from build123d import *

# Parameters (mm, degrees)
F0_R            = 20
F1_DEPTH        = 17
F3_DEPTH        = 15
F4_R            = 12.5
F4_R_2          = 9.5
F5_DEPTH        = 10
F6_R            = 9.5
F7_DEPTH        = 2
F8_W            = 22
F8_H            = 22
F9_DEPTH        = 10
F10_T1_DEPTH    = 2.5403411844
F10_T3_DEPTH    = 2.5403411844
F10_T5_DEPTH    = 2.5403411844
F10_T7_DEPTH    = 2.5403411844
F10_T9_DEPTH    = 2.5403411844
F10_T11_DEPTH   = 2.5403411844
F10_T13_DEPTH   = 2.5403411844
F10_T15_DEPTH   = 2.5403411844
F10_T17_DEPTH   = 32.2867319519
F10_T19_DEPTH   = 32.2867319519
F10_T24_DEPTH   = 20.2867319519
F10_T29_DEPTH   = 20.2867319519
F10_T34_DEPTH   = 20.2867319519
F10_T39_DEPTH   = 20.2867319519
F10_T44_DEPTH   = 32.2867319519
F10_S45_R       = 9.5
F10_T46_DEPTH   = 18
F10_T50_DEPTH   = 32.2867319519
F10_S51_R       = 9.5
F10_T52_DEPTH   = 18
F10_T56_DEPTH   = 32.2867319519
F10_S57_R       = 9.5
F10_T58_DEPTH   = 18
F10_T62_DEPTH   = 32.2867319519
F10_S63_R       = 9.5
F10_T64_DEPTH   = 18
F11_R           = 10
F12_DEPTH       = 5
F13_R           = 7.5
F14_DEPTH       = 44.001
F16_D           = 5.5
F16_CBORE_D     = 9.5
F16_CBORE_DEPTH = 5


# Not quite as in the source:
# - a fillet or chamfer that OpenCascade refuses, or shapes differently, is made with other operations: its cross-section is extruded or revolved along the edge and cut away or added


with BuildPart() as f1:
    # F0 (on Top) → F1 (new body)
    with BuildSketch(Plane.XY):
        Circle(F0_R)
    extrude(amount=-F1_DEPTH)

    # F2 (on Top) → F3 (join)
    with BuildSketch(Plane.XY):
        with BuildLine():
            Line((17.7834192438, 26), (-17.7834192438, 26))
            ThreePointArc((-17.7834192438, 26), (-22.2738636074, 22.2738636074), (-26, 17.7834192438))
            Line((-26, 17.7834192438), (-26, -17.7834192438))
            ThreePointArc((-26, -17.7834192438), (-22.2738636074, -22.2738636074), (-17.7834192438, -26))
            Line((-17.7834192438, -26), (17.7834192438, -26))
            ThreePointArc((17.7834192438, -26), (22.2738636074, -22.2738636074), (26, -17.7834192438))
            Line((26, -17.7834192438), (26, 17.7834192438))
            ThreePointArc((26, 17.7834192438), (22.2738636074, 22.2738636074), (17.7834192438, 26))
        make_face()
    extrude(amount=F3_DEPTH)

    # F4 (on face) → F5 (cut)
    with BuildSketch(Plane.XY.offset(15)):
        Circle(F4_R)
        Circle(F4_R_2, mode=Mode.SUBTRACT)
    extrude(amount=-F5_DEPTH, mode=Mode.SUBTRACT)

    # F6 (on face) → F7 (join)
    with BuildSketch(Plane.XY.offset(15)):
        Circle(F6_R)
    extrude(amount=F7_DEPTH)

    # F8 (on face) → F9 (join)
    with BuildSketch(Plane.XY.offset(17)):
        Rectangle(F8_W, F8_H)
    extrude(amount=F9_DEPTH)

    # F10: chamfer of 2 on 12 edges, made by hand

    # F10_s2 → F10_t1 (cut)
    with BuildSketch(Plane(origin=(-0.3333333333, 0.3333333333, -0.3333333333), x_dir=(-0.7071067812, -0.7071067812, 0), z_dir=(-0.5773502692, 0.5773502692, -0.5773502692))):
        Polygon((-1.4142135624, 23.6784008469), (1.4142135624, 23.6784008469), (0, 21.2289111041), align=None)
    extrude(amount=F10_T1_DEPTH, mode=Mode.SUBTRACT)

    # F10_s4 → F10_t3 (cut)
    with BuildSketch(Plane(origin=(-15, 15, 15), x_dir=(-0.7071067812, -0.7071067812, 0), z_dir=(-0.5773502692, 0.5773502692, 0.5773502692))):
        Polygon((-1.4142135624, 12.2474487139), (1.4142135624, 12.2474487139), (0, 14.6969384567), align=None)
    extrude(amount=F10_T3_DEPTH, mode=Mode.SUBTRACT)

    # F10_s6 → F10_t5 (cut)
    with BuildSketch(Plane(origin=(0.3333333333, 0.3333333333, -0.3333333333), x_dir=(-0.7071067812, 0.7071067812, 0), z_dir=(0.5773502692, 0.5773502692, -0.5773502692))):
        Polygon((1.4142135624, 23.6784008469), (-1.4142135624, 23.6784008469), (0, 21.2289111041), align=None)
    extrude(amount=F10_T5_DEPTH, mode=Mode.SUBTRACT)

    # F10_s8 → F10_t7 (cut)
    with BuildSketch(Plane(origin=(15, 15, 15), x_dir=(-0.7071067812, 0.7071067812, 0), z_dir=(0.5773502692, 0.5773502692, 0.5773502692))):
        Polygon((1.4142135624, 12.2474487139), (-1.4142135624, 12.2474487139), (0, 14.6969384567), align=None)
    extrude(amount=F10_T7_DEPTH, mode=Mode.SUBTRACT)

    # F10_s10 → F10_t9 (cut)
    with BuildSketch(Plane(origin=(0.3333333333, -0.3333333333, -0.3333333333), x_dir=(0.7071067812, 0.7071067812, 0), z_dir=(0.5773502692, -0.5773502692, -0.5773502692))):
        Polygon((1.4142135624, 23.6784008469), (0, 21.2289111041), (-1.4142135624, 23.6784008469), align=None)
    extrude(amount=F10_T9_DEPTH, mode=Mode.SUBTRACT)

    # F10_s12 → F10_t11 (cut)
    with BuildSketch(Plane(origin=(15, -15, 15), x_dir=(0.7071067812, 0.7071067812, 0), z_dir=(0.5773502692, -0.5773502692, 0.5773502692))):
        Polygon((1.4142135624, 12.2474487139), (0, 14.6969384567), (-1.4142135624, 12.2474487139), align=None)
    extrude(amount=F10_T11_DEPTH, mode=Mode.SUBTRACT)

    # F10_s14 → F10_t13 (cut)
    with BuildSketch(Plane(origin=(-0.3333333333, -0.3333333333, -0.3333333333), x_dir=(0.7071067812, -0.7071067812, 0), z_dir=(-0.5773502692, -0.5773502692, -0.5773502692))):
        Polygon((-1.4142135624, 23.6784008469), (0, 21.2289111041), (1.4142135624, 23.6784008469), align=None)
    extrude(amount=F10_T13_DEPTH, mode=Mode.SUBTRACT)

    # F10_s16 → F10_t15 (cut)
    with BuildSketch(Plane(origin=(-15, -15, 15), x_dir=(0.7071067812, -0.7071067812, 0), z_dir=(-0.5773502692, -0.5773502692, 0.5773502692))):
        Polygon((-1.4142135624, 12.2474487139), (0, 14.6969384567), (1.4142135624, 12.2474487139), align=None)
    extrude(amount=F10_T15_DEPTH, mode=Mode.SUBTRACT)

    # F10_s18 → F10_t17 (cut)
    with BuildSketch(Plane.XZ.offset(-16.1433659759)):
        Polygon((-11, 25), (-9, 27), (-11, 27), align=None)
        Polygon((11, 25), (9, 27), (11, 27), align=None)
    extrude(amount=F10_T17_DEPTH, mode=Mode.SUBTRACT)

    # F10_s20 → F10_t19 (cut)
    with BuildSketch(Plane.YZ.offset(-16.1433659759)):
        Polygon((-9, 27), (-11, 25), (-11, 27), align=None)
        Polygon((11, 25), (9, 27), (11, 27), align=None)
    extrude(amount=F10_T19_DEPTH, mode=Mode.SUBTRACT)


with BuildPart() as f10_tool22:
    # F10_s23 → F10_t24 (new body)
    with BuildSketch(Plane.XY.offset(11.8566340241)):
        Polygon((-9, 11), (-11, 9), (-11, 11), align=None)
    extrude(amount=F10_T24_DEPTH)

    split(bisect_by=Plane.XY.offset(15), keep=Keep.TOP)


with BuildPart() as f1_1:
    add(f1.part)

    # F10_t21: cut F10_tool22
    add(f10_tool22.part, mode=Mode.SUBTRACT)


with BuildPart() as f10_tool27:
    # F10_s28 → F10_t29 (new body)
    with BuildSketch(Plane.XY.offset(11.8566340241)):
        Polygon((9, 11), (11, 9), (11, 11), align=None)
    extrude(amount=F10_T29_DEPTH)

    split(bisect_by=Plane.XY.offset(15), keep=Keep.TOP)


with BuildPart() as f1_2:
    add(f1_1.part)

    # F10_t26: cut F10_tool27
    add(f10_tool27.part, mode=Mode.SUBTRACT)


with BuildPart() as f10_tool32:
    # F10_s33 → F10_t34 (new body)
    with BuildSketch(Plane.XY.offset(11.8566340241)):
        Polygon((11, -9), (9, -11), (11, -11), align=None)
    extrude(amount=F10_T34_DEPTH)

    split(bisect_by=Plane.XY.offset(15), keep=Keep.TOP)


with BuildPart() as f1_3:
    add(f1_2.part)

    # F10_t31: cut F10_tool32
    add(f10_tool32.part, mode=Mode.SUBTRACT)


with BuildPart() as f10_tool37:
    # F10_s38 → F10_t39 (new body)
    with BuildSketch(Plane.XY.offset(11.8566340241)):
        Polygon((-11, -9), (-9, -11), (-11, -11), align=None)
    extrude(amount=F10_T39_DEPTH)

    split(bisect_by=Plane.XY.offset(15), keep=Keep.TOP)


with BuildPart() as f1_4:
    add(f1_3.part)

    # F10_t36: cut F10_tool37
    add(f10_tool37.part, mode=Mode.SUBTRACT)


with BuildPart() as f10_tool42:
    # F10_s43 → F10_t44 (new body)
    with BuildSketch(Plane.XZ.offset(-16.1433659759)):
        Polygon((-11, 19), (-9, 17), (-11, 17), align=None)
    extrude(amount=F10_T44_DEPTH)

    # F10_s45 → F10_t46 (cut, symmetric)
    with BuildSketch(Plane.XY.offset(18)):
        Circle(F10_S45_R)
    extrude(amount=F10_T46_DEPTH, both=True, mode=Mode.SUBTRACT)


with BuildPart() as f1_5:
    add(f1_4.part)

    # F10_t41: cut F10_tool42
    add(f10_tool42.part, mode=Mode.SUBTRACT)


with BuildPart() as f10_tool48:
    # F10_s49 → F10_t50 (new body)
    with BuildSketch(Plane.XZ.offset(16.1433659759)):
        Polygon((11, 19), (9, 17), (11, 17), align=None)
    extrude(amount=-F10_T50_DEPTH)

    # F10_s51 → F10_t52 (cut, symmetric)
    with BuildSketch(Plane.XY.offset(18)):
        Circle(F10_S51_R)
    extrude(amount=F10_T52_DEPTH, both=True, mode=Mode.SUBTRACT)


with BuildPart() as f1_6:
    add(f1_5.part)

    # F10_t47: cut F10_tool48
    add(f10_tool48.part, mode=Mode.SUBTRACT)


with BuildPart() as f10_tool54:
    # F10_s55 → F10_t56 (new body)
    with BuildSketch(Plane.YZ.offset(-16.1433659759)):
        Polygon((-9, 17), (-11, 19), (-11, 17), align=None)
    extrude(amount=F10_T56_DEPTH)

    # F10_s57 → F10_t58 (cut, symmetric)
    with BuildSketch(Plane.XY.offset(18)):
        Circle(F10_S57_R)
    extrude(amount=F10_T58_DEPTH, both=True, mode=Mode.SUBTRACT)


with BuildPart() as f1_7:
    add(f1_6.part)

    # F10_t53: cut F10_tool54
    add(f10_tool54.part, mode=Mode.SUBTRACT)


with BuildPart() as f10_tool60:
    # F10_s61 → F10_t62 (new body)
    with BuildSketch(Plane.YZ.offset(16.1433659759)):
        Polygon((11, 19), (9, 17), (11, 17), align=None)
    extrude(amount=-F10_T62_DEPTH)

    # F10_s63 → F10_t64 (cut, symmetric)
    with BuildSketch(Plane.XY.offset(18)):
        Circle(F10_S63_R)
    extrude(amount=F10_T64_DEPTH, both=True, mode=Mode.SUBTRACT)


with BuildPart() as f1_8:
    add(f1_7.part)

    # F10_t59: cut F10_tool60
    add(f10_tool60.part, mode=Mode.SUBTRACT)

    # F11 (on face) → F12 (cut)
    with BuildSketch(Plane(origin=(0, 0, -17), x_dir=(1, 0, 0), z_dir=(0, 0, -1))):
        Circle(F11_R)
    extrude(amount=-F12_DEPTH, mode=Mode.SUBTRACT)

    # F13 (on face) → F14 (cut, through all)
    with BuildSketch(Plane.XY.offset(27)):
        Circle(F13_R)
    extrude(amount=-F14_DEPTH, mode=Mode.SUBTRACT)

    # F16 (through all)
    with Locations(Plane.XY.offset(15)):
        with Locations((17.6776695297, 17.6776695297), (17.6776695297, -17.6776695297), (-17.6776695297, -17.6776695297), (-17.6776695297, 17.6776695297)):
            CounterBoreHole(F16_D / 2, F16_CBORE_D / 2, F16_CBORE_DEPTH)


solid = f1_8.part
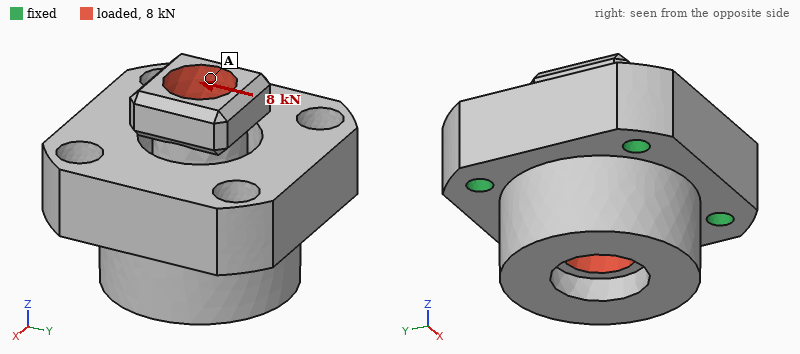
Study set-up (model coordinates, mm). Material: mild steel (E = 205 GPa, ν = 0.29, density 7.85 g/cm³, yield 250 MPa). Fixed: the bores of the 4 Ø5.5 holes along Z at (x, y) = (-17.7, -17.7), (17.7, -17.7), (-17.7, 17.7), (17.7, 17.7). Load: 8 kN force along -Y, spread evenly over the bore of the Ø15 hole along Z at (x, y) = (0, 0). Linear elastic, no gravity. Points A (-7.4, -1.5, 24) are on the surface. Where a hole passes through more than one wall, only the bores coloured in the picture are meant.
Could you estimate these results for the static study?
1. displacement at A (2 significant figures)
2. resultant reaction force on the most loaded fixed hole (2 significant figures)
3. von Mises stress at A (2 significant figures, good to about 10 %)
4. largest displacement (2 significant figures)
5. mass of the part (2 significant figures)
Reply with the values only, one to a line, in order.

23 µm
2.1 kN
18 MPa
27 µm
410 g
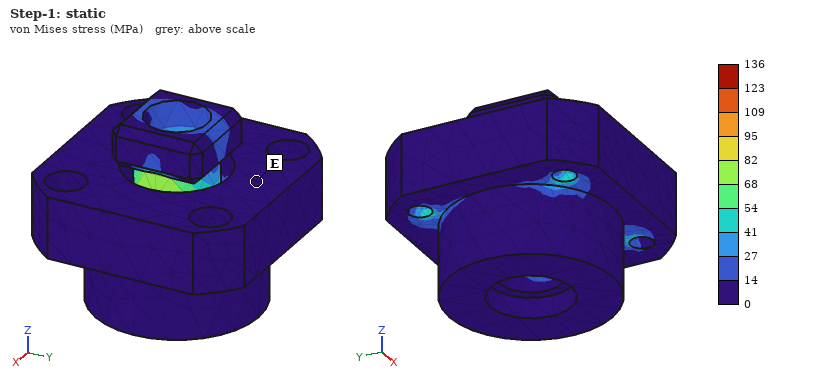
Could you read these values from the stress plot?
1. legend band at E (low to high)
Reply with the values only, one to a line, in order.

0 to 14 MPa
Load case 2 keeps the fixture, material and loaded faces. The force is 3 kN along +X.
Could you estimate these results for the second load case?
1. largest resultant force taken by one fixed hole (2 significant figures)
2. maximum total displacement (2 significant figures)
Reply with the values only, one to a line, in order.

780 N
10 µm
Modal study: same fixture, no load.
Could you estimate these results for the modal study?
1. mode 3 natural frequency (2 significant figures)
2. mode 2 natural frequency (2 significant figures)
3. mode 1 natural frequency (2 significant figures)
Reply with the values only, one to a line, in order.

20 kHz
12 kHz
12 kHz
